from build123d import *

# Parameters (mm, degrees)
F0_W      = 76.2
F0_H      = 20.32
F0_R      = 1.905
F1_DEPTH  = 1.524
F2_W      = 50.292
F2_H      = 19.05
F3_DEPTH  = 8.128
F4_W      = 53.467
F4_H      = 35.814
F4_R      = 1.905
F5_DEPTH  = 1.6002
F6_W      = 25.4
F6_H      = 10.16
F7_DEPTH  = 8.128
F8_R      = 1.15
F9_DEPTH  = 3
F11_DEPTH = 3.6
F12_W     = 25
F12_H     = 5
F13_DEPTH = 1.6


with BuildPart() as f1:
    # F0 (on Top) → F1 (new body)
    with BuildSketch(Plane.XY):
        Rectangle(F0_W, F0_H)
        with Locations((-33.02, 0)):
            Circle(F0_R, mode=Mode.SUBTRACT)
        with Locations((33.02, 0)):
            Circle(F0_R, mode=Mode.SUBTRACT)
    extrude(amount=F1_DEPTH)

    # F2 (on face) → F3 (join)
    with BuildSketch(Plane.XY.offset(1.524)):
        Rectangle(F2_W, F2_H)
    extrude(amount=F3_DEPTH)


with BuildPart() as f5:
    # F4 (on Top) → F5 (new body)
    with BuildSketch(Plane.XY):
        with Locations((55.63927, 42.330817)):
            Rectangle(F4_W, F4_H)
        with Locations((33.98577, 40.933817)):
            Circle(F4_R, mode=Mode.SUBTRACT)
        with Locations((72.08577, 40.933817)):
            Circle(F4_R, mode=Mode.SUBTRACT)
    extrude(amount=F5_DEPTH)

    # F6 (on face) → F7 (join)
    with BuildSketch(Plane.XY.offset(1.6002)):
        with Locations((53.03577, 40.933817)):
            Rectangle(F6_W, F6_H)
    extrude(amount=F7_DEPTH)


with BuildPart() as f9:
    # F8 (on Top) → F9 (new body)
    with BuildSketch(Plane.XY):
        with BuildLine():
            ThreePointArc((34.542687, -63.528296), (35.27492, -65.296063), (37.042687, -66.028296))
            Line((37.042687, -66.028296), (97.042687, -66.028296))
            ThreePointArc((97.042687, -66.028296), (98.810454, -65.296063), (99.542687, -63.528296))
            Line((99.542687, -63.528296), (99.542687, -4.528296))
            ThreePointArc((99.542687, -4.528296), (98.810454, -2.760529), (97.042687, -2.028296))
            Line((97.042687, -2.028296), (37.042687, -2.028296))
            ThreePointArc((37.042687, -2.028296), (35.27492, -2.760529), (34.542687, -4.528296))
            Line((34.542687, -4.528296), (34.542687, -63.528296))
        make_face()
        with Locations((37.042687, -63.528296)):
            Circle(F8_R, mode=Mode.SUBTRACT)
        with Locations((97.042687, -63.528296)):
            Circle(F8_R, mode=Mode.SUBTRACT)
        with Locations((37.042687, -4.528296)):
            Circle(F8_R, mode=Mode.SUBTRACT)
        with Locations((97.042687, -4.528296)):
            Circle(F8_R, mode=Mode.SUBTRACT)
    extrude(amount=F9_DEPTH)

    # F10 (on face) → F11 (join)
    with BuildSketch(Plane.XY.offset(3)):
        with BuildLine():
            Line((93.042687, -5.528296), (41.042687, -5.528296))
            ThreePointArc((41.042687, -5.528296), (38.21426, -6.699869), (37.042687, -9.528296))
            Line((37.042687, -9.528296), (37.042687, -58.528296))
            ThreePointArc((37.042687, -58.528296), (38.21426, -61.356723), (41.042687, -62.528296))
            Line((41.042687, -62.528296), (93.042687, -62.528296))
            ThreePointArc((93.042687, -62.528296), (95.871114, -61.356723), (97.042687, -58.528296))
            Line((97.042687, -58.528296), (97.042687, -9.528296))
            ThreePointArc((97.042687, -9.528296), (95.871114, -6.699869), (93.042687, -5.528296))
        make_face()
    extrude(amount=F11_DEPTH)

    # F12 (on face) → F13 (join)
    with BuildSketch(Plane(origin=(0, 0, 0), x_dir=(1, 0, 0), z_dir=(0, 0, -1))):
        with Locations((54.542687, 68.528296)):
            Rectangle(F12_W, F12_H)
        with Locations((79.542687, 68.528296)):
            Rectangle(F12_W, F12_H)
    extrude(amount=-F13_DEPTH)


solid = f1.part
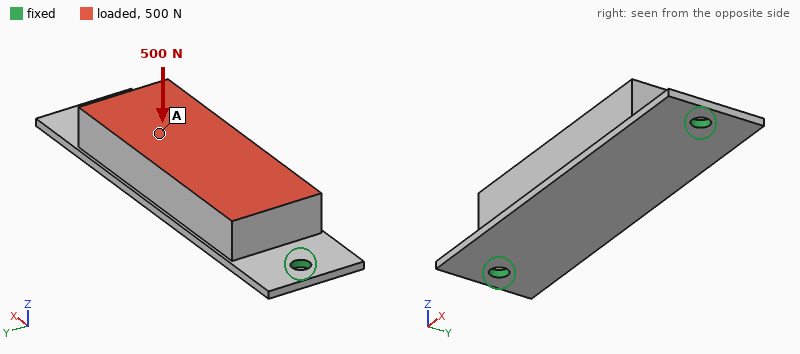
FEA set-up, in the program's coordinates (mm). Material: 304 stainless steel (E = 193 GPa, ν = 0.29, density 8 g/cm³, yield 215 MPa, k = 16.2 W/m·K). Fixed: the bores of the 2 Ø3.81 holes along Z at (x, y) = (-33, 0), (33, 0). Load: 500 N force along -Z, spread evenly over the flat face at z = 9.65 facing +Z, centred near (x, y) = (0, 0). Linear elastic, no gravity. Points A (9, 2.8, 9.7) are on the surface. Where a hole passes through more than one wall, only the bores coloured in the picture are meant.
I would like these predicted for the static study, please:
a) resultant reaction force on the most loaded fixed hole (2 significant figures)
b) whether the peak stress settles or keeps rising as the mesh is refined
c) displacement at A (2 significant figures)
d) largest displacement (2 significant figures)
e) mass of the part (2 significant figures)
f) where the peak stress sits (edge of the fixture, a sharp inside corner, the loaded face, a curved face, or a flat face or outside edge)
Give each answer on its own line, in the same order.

380 N
keeps rising
15 µm
16 µm
81 g
edge of the fixture
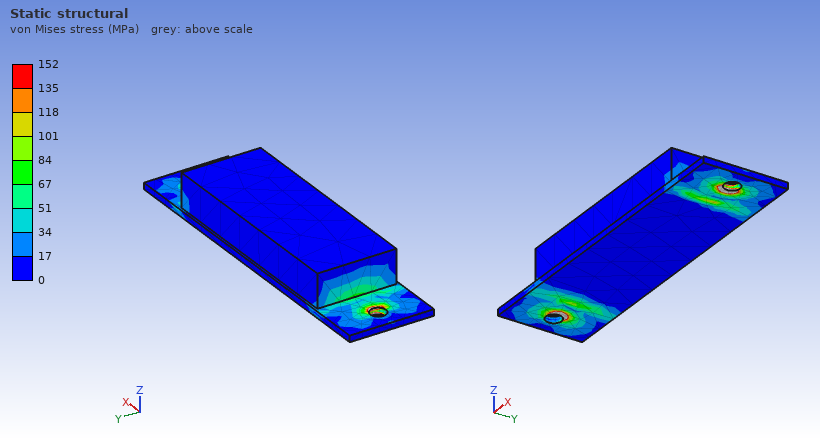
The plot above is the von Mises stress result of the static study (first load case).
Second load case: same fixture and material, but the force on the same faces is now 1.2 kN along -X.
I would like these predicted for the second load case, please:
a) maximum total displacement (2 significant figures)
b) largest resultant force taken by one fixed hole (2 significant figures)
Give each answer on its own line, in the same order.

8.9 µm
630 N
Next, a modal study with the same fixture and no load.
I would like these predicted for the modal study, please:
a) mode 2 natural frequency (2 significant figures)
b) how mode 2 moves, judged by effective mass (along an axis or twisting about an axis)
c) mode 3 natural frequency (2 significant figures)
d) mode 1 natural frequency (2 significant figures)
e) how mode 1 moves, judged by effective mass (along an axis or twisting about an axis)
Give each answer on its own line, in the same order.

3400 Hz
along Z
6600 Hz
2100 Hz
along Y
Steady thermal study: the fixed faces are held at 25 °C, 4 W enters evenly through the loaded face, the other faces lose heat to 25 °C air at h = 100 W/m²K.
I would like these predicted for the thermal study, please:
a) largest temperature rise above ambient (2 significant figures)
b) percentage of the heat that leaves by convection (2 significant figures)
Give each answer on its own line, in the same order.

15 K
81 %
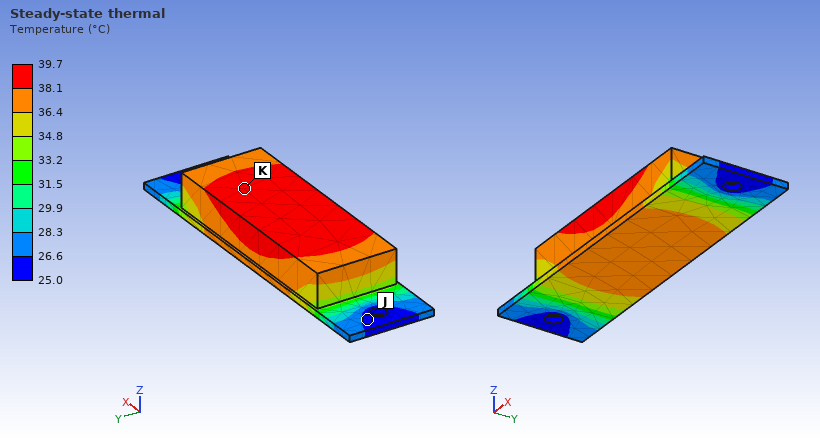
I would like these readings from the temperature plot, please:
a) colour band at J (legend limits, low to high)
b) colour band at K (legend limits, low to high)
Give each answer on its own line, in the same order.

25.0 to 26.6 °C
38.1 to 39.7 °C
